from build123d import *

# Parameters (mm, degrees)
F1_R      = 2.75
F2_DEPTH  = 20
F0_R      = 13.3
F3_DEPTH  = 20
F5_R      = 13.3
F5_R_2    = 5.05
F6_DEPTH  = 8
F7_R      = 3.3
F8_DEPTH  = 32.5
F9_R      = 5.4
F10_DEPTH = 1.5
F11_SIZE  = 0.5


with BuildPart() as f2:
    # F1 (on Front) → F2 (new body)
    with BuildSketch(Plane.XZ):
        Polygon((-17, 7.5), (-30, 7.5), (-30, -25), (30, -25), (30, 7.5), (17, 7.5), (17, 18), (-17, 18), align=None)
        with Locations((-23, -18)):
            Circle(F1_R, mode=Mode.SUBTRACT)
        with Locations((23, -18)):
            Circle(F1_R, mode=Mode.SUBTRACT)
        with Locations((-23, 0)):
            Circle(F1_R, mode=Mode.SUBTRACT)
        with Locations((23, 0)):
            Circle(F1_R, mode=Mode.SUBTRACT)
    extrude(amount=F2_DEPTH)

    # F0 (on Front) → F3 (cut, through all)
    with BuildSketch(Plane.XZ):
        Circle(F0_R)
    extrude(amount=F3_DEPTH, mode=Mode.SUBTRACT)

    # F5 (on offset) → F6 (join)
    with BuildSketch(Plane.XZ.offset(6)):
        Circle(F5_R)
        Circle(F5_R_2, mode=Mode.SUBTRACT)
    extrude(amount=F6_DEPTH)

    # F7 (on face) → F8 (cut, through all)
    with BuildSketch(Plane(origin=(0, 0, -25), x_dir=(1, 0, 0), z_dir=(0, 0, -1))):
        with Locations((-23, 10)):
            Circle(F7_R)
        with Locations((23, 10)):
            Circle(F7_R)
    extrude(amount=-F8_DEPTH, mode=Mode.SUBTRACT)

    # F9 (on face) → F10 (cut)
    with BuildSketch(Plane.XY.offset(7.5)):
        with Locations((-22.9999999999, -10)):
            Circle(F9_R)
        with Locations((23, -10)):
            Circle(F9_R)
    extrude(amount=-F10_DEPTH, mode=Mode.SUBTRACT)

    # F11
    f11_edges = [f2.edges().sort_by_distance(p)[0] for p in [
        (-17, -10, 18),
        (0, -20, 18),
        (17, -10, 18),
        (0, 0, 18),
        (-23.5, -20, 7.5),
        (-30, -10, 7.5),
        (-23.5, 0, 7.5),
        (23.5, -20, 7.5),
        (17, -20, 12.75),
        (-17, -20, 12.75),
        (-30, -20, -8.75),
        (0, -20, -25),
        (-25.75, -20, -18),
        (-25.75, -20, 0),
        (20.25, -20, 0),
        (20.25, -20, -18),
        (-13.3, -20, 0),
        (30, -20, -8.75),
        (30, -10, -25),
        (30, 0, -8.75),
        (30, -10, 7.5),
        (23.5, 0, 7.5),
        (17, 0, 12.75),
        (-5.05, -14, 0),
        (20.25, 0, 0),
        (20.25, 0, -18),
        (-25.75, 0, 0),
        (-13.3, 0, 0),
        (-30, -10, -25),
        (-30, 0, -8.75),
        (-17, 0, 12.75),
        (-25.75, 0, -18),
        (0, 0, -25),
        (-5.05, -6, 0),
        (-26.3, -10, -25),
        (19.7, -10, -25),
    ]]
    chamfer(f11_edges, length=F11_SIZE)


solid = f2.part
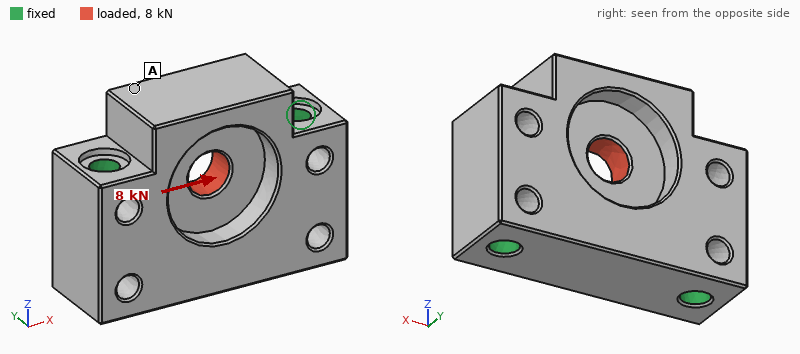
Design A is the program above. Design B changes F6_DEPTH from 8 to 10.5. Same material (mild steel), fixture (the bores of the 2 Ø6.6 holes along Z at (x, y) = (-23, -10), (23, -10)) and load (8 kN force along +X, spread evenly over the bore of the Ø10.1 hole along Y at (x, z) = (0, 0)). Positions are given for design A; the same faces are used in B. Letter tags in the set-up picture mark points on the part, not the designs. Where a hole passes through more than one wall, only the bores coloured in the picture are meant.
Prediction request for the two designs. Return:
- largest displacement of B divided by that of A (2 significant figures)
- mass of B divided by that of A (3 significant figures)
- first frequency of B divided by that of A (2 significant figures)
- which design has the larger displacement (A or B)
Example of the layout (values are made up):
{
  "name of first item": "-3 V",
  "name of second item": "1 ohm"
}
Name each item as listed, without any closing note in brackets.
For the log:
{
  "largest displacement of B divided by that of A": "0.83",
  "mass of B divided by that of A": "1.03",
  "first frequency of B divided by that of A": "1.0",
  "which design has the larger displacement": "A"
}
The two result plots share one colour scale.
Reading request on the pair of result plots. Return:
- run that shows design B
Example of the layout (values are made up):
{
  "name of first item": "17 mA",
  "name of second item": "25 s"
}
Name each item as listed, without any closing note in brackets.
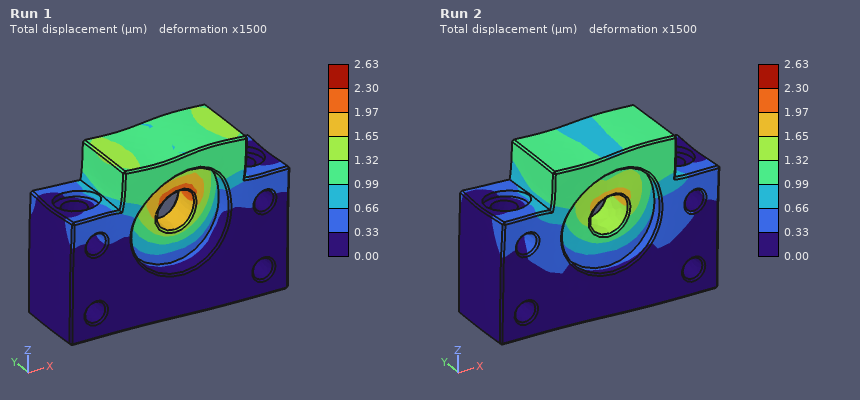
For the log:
{
  "run that shows design B": "Run 2"
}
